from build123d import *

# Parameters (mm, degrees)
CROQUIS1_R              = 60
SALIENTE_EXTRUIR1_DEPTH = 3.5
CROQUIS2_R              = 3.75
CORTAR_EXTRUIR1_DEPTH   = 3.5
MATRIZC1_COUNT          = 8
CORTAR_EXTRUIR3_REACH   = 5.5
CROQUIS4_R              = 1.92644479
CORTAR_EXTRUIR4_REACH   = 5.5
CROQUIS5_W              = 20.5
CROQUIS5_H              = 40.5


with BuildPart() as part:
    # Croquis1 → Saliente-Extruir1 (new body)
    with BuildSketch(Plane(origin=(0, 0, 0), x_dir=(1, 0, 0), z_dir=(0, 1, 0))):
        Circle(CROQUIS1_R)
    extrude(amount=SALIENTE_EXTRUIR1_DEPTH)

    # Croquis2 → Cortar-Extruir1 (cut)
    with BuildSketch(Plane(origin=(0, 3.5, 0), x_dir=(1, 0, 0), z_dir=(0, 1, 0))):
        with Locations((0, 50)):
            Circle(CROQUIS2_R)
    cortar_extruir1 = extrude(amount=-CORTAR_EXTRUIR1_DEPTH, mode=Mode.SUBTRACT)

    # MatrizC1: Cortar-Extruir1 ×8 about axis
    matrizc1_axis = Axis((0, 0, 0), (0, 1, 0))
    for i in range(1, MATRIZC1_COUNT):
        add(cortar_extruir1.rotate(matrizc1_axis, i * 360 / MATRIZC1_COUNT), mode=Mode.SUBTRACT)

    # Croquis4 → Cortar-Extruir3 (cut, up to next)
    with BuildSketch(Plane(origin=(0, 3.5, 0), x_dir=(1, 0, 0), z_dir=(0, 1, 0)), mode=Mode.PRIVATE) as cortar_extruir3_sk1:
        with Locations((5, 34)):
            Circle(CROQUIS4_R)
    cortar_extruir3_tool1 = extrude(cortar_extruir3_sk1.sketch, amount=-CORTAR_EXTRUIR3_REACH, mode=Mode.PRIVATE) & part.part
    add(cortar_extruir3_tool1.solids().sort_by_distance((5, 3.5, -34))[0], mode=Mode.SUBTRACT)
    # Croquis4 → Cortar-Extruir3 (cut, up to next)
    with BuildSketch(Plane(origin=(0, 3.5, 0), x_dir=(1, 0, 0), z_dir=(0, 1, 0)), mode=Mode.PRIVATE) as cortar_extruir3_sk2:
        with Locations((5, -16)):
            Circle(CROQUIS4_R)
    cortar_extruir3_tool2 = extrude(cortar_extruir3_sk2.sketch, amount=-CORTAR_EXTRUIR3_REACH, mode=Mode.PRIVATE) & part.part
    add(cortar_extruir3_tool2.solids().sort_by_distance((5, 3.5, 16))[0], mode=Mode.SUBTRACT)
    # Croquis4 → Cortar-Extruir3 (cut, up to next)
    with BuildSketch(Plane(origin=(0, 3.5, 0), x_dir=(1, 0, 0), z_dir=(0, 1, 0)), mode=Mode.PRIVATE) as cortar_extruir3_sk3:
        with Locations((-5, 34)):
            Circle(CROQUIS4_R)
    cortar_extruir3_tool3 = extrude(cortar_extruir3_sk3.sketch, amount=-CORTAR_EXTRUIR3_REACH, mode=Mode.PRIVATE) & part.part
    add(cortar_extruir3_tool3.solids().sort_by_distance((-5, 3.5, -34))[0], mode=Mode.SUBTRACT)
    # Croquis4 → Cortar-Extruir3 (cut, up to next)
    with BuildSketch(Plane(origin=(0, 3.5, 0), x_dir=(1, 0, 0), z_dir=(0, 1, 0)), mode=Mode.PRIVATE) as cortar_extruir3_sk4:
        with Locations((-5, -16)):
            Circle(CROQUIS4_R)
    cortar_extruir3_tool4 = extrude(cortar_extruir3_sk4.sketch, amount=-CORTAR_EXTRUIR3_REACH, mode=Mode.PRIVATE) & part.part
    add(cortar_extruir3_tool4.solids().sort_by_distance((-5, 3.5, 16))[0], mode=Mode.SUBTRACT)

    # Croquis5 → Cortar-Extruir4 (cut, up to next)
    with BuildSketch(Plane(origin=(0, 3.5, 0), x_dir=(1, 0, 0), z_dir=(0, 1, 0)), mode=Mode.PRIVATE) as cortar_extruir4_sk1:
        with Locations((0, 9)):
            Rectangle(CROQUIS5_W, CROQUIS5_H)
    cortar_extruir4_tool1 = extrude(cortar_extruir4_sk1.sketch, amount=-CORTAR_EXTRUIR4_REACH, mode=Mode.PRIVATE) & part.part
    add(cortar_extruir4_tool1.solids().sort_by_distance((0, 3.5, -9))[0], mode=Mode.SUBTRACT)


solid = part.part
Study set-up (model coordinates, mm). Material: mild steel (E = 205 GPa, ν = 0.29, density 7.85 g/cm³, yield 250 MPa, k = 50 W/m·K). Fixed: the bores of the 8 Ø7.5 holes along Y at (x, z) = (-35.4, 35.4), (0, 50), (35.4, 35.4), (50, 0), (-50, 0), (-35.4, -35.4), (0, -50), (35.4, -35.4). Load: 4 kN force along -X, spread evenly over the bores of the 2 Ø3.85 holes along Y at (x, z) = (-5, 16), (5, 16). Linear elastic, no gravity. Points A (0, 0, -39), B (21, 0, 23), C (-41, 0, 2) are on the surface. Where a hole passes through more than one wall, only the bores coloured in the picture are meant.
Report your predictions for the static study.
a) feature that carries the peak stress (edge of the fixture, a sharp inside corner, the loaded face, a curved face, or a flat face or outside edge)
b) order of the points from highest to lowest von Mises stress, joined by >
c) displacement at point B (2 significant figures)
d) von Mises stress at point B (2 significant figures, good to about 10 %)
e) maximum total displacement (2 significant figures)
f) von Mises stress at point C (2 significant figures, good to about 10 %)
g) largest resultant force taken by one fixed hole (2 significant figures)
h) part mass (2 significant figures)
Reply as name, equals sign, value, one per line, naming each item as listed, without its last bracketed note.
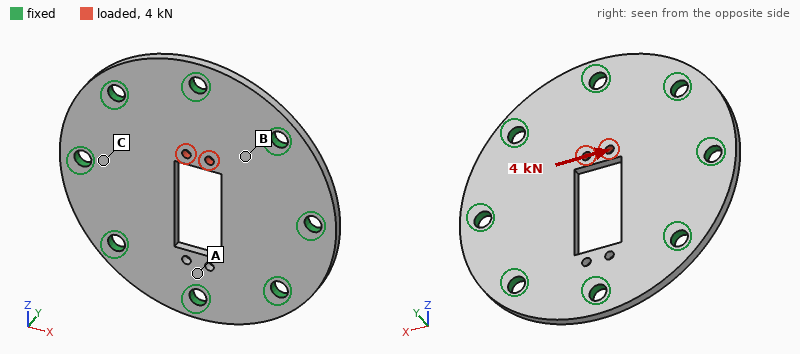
feature that carries the peak stress = the loaded face
order of the points from highest to lowest von Mises stress, joined by > = B > C > A
displacement at point B = 1.7 µm
von Mises stress at point B = 22 MPa
maximum total displacement = 5.7 µm
von Mises stress at point C = 12 MPa
largest resultant force taken by one fixed hole = 1.2 kN
part mass = 280 g
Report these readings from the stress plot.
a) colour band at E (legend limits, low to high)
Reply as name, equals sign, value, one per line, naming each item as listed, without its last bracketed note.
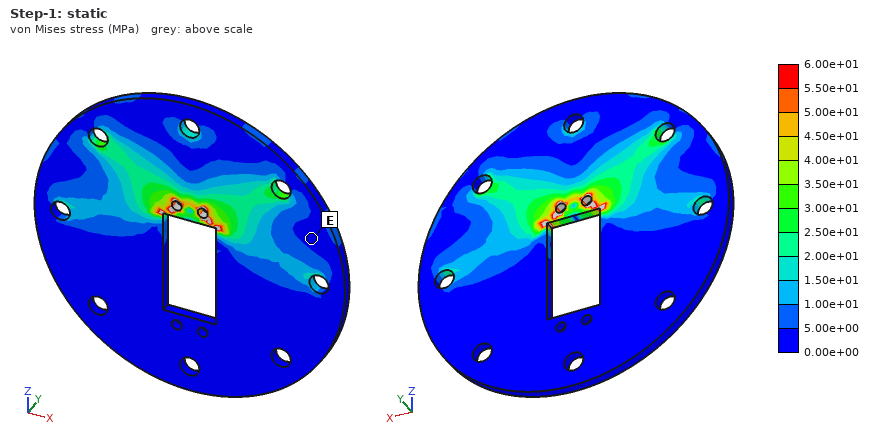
colour band at E = 0.00e+00 to 5.00e+00 MPa
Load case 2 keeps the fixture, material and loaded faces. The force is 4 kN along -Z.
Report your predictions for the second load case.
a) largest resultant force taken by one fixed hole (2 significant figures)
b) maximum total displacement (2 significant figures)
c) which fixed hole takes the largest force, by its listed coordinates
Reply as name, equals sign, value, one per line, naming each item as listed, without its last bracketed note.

largest resultant force taken by one fixed hole = 1.8 kN
maximum total displacement = 6.3 µm
which fixed hole takes the largest force, by its listed coordinates = (0, 50)
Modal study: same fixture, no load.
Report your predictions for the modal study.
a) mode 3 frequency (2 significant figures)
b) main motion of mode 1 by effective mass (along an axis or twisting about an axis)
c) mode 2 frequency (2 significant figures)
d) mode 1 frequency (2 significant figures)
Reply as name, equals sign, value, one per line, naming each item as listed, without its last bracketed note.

mode 3 frequency = 7200 Hz
main motion of mode 1 by effective mass = along Y
mode 2 frequency = 5300 Hz
mode 1 frequency = 3800 Hz
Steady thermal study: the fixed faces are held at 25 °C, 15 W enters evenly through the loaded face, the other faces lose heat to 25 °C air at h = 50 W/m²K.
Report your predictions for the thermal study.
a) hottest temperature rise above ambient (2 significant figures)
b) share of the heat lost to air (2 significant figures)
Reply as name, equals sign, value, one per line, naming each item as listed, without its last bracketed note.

hottest temperature rise above ambient = 44 K
share of the heat lost to air = 27 %
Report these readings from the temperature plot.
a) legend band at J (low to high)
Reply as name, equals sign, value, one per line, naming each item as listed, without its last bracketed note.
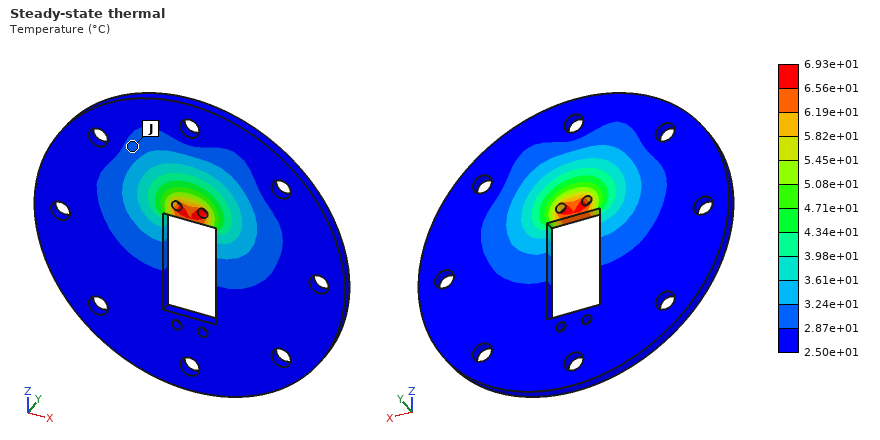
legend band at J = 2.87e+01 to 3.24e+01 °C
